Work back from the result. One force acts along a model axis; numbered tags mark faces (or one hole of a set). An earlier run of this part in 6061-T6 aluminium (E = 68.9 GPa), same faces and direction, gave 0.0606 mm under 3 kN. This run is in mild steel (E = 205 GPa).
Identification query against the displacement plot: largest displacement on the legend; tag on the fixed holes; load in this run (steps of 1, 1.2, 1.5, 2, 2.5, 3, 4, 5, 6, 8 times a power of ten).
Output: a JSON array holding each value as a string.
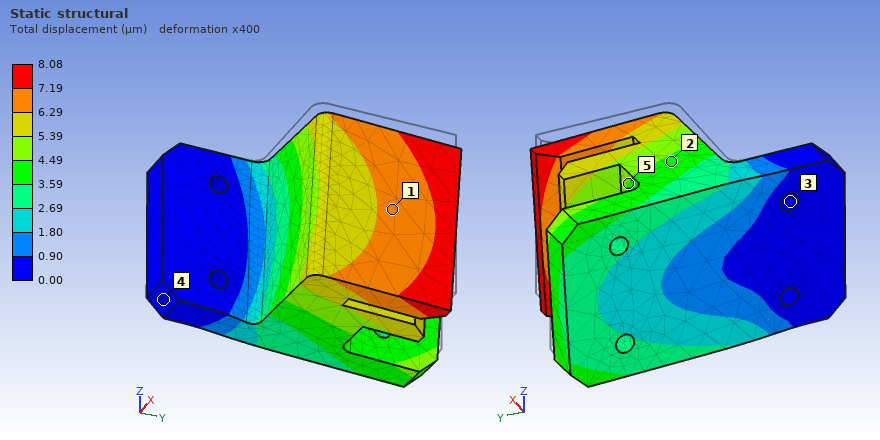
["8.08 µm", "3", "1.2 kN"]
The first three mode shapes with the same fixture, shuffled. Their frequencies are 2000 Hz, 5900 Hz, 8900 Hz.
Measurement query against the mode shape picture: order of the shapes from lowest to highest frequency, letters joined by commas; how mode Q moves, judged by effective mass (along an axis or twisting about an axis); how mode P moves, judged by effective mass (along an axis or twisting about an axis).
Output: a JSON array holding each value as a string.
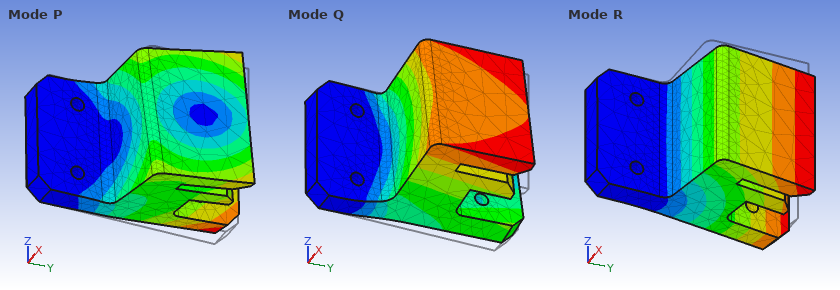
["R, Q, P", "along Z", "along Z"]
